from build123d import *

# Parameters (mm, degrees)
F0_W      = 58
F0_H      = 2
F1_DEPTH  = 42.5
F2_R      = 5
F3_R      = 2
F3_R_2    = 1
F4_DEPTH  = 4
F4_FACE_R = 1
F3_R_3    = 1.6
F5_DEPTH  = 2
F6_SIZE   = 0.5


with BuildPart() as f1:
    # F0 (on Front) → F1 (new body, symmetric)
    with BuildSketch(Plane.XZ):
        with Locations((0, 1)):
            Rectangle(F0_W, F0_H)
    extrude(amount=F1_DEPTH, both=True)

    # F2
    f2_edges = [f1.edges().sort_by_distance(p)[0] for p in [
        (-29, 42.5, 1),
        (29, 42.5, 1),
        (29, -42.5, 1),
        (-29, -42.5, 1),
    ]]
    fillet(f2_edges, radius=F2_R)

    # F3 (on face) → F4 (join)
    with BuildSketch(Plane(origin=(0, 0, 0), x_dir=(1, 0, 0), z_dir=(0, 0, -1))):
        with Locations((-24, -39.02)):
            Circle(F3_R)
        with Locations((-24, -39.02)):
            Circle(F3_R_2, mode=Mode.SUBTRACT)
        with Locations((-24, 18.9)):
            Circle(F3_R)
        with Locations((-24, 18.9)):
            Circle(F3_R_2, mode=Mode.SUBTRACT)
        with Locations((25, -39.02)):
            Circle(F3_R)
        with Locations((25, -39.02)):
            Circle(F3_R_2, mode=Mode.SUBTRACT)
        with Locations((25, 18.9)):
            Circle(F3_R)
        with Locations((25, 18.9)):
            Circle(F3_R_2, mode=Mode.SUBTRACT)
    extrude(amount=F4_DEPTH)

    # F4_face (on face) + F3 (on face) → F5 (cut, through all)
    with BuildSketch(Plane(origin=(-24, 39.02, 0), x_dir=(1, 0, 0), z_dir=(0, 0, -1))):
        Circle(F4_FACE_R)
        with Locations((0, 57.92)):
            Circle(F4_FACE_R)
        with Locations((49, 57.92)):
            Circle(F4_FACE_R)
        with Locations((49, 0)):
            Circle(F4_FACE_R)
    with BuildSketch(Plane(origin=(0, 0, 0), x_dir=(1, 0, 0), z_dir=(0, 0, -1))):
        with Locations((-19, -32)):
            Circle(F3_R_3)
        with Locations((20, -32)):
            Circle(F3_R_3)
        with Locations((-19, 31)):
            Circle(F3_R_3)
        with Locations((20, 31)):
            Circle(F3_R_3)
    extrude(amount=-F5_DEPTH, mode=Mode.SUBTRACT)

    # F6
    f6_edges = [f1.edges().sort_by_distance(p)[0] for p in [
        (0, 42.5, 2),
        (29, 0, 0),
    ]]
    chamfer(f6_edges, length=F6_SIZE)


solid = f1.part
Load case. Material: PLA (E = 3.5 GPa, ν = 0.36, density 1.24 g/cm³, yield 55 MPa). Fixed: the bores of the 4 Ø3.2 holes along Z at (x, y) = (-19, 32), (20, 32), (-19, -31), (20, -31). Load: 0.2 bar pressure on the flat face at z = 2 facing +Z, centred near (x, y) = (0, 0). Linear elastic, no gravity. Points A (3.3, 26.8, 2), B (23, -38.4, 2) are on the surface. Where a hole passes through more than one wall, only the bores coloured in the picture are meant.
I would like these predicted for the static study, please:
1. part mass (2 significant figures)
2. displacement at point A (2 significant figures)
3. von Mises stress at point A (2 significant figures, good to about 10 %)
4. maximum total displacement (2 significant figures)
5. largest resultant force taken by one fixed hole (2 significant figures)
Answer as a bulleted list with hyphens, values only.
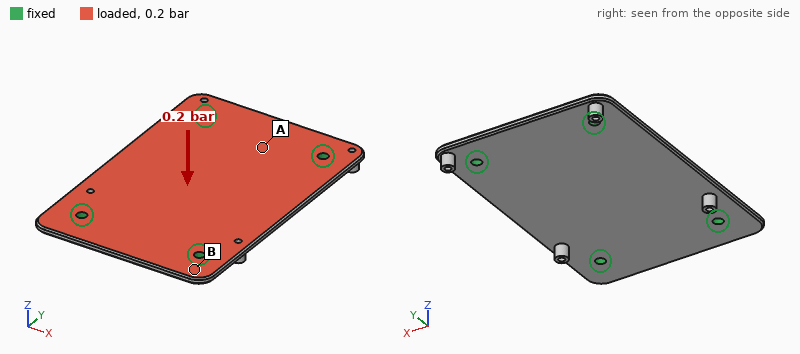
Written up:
- 12 g
- 0.13 mm
- 3.1 MPa
- 0.42 mm
- 24 N
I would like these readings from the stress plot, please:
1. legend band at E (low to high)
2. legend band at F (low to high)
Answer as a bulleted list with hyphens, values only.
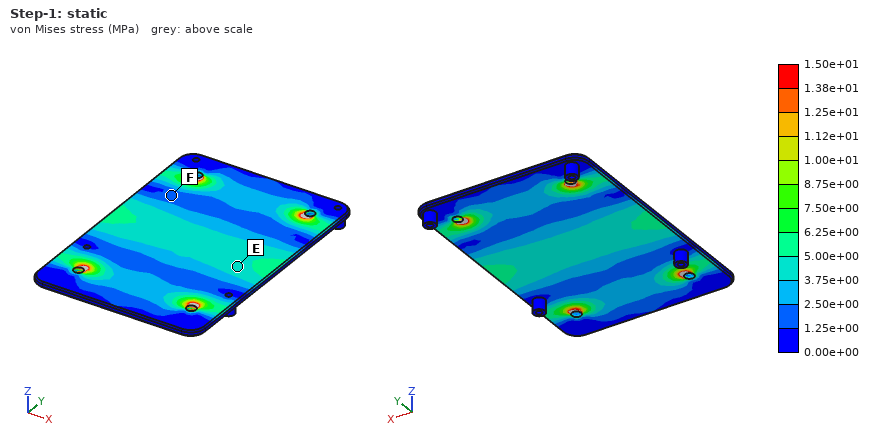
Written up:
- 3.75e+00 to 5.00e+00 MPa
- 1.25e+00 to 2.50e+00 MPa
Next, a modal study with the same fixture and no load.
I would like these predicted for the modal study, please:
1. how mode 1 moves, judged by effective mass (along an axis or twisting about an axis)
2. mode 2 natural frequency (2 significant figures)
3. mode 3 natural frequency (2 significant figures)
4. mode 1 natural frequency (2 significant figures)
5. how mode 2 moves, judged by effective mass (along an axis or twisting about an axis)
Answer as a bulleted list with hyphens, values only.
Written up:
- along Z
- 1100 Hz
- 1600 Hz
- 800 Hz
- twisting about Y
